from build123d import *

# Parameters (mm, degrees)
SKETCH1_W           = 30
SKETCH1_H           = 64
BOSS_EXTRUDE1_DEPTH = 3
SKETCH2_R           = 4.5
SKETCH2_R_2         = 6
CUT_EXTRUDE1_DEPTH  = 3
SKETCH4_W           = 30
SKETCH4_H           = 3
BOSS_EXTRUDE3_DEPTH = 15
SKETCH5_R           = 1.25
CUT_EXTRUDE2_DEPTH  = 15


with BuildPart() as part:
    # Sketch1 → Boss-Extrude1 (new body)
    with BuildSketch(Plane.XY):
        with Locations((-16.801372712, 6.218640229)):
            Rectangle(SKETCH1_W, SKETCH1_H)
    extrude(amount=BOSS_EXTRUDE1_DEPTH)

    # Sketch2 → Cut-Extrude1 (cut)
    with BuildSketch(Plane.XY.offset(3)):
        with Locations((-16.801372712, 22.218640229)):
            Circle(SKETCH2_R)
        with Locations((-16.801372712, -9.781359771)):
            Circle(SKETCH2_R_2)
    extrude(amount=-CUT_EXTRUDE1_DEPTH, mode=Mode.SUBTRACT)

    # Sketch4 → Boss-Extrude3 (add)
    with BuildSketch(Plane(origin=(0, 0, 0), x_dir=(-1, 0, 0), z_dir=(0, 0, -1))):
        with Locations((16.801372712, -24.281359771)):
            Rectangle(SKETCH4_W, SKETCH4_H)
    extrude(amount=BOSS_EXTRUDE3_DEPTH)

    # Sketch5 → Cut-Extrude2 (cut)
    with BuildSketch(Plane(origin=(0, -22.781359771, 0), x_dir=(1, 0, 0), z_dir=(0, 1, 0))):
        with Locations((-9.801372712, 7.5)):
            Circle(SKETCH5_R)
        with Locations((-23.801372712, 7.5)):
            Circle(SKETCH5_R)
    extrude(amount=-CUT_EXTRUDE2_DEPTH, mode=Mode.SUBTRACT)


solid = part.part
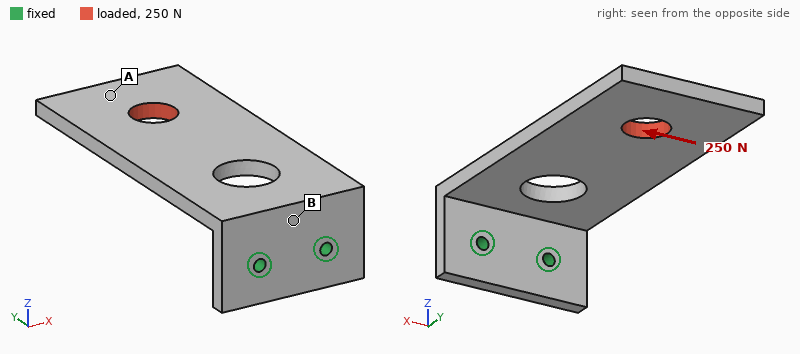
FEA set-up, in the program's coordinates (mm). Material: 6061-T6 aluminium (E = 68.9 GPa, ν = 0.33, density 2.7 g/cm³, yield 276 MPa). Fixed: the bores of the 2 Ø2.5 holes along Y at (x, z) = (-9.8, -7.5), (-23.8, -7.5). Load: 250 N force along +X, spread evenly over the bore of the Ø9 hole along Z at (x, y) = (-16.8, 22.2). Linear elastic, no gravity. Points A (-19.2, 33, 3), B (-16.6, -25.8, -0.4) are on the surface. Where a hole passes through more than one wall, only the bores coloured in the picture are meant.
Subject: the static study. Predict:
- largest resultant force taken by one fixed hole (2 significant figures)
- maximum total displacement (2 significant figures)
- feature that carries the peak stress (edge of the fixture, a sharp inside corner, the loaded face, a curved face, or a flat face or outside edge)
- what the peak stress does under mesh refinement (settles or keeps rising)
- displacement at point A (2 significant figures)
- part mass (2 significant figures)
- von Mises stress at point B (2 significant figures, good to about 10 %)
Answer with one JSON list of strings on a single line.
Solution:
["680 N", "0.38 mm", "edge of the fixture", "keeps rising", "0.32 mm", "18 g", "81 MPa"]
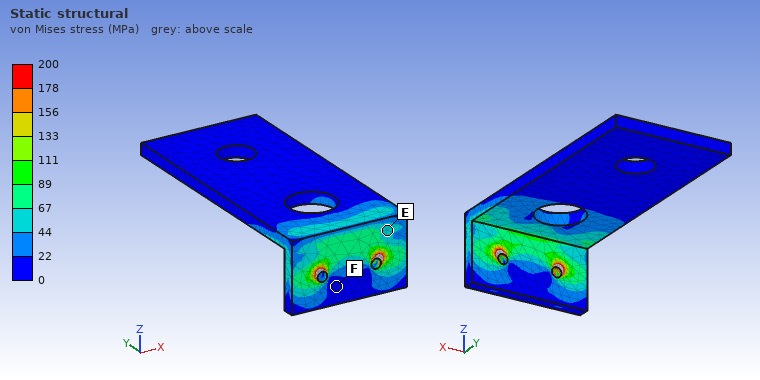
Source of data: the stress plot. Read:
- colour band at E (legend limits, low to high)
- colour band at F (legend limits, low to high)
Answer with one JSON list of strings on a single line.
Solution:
["44 to 67 MPa", "0 to 22 MPa"]
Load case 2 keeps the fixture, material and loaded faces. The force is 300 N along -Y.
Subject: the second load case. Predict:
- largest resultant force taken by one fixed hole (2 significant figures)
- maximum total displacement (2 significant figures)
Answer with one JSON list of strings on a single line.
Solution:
["150 N", "0.18 mm"]
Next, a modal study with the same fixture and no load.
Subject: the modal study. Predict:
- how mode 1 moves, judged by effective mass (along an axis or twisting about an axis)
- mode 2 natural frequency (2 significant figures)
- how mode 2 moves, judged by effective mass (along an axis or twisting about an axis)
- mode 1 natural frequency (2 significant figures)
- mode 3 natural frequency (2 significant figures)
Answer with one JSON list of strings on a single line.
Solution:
["along Z", "1600 Hz", "along X", "490 Hz", "2500 Hz"]
